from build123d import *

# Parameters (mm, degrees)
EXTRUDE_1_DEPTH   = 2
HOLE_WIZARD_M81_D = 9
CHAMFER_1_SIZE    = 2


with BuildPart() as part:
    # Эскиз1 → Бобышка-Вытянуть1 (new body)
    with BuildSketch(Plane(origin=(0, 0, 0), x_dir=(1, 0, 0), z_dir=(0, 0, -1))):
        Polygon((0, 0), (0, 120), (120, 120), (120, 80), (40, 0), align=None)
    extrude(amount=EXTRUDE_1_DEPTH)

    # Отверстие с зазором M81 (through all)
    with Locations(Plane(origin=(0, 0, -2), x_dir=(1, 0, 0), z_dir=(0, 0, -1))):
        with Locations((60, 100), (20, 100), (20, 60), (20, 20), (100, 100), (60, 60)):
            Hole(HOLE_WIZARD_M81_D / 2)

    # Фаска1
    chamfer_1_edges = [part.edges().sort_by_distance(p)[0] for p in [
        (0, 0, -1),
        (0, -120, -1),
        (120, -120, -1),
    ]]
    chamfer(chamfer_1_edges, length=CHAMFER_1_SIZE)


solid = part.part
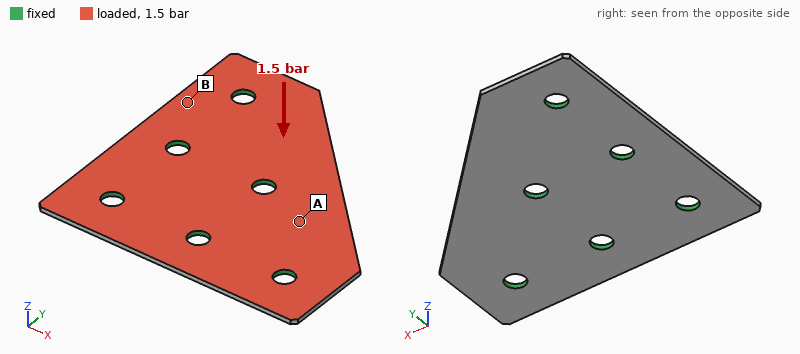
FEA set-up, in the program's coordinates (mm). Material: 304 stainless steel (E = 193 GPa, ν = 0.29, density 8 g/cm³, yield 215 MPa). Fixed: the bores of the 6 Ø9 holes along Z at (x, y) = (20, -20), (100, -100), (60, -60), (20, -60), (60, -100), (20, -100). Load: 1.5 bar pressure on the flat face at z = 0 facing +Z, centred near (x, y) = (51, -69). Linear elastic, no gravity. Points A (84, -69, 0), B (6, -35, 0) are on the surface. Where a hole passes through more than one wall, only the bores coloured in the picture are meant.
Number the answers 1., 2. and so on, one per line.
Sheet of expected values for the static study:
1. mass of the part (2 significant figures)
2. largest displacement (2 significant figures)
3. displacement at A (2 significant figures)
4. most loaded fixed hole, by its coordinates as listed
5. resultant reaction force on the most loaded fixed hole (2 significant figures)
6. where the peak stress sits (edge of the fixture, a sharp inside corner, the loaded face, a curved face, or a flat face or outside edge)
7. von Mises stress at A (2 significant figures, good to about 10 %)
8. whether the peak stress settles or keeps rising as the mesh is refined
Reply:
1. 170 g
2. 99 µm
3. 39 µm
4. (60, -60)
5. 370 N
6. edge of the fixture
7. 31 MPa
8. keeps rising
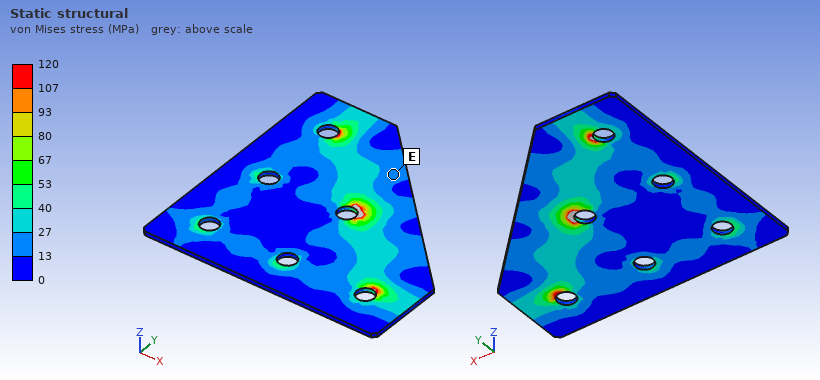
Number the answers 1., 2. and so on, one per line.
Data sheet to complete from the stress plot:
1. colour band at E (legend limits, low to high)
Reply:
1. 13 to 27 MPa
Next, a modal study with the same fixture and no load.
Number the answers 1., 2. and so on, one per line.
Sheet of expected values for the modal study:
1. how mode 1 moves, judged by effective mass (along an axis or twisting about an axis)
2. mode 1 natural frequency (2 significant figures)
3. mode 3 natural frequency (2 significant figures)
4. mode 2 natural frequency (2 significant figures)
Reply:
1. along Z
2. 2000 Hz
3. 3700 Hz
4. 2300 Hz
